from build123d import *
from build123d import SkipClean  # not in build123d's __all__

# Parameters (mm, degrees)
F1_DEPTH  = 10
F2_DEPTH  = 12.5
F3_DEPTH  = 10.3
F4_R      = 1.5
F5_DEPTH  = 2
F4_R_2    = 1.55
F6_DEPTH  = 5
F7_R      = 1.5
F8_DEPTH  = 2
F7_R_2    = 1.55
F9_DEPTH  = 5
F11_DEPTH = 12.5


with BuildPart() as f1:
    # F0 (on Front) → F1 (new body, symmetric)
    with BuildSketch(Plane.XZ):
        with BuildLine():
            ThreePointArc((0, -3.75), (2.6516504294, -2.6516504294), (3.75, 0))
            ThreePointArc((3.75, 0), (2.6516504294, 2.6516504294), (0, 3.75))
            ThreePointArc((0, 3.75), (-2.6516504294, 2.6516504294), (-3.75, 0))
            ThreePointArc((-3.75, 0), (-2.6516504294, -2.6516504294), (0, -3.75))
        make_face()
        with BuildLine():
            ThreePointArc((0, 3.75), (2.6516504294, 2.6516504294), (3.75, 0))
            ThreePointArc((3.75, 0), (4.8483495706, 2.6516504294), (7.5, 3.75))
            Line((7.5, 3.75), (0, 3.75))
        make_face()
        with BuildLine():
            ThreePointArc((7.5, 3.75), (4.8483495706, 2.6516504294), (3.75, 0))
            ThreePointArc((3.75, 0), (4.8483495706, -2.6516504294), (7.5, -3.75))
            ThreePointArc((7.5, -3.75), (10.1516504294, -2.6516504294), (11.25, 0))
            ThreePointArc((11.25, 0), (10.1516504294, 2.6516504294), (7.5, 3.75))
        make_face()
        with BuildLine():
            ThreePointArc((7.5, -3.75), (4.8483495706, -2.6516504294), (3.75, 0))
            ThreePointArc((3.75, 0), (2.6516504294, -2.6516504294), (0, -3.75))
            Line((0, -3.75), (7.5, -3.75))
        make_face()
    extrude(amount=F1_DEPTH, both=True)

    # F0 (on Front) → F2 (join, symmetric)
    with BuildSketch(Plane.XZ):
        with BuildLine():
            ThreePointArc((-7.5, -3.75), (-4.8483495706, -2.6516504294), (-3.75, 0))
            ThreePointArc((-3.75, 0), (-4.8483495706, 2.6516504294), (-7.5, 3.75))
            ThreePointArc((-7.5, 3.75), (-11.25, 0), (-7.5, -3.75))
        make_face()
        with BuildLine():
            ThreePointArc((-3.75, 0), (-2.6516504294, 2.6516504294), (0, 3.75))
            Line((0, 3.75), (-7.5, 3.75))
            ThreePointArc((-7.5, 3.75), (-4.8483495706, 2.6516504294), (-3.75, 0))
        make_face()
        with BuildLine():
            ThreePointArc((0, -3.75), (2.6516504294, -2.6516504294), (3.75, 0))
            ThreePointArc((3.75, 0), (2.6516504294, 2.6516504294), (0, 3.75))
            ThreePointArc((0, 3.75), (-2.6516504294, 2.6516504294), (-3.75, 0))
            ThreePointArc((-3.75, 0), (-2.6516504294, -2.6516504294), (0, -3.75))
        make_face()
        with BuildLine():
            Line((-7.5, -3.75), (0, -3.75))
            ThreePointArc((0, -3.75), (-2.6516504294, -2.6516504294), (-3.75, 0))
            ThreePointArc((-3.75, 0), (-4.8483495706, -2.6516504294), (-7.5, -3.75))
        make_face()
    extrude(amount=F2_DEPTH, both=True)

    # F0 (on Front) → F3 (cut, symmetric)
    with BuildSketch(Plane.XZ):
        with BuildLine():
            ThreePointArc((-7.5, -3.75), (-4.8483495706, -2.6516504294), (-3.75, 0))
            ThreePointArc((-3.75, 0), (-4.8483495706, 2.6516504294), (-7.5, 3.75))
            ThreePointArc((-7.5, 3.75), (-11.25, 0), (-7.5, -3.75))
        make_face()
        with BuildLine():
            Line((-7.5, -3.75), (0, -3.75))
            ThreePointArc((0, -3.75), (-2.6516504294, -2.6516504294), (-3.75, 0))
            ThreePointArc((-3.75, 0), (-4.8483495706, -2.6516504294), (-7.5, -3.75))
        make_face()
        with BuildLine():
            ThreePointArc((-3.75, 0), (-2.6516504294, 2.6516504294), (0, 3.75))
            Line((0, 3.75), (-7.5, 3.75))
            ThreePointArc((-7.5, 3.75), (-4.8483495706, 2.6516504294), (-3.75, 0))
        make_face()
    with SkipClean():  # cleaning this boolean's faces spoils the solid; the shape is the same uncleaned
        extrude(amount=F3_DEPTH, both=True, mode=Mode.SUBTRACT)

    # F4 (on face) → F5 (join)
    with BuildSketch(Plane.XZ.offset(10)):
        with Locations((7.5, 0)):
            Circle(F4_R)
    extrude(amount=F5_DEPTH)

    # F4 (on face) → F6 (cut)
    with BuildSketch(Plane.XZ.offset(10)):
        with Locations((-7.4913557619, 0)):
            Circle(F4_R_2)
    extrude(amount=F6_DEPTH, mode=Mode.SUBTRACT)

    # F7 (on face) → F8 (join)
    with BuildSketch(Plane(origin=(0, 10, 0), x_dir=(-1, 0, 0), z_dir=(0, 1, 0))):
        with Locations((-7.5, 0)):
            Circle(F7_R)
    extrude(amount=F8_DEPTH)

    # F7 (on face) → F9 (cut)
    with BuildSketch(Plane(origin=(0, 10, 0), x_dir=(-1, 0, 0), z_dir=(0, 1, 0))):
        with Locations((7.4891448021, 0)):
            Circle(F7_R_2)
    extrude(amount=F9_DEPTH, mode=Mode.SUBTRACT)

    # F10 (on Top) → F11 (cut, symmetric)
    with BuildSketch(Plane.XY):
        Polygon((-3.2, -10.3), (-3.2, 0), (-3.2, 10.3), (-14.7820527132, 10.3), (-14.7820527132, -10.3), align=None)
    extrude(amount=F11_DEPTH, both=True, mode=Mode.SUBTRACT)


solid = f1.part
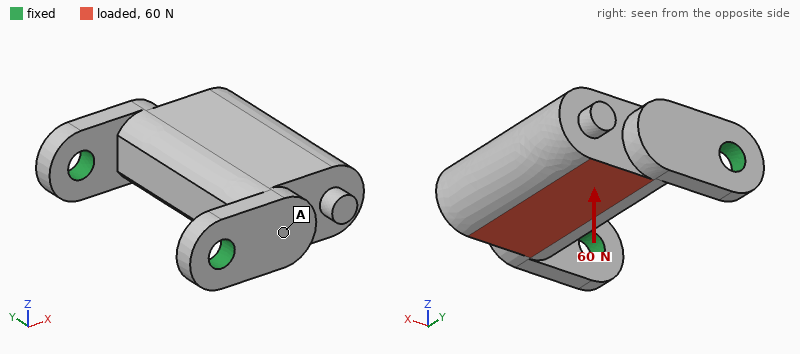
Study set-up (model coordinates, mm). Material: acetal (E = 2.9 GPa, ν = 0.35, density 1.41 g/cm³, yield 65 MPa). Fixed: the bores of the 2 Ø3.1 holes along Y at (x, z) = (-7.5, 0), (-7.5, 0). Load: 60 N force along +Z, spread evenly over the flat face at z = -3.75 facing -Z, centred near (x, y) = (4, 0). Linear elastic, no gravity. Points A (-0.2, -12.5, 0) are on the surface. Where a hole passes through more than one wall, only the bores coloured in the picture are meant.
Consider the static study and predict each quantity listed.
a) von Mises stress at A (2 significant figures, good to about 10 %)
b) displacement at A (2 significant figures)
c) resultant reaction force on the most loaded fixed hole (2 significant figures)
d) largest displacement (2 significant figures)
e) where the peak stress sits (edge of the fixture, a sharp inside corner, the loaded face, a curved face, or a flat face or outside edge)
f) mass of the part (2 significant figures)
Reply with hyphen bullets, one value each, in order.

- 3.8 MPa
- 0.056 mm
- 30 N
- 0.20 mm
- edge of the fixture
- 3.4 g
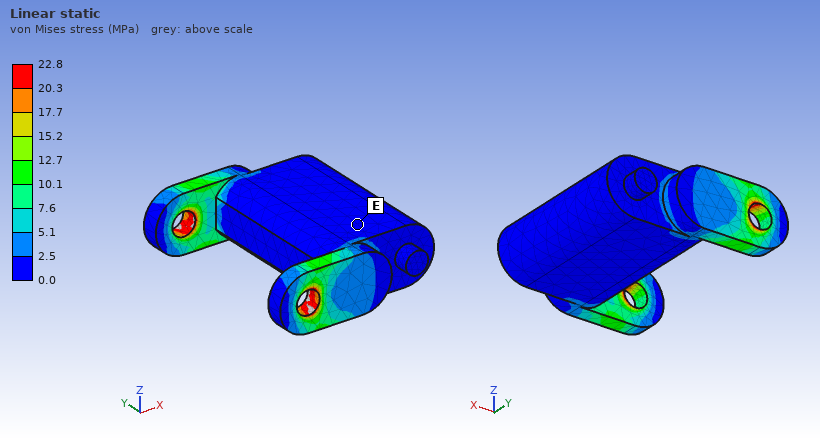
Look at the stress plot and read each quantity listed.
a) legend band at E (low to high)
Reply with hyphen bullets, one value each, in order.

- 0.0 to 2.5 MPa
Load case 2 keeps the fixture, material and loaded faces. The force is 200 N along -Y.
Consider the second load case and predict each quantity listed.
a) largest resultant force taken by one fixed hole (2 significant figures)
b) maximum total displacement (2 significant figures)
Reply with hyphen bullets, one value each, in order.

- 130 N
- 0.11 mm
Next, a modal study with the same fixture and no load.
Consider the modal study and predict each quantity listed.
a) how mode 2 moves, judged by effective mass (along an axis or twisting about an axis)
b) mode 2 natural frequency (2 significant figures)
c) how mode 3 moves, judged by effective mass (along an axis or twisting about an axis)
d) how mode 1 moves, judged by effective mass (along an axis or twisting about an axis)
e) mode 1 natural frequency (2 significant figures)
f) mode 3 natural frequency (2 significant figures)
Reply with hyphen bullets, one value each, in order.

- along Y
- 4400 Hz
- twisting about X
- along Z
- 1900 Hz
- 6500 Hz
